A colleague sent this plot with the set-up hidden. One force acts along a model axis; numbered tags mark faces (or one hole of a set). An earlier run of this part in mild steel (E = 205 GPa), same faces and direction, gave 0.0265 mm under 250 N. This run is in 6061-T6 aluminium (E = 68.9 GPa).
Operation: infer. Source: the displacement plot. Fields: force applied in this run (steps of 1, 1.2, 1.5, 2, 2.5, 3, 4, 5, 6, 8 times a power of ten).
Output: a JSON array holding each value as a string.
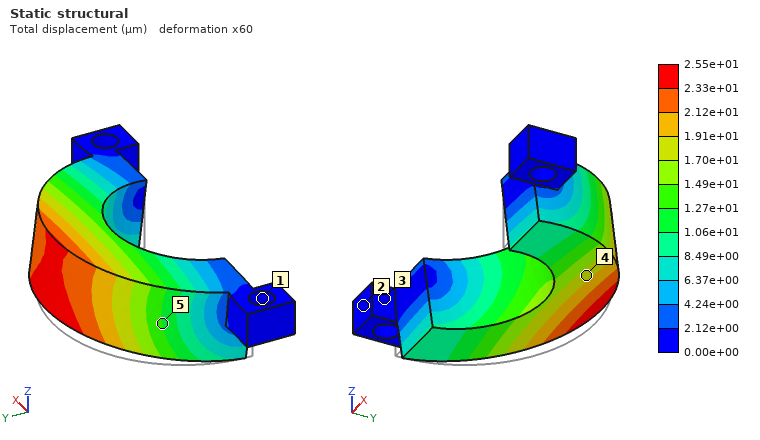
["80 N"]
